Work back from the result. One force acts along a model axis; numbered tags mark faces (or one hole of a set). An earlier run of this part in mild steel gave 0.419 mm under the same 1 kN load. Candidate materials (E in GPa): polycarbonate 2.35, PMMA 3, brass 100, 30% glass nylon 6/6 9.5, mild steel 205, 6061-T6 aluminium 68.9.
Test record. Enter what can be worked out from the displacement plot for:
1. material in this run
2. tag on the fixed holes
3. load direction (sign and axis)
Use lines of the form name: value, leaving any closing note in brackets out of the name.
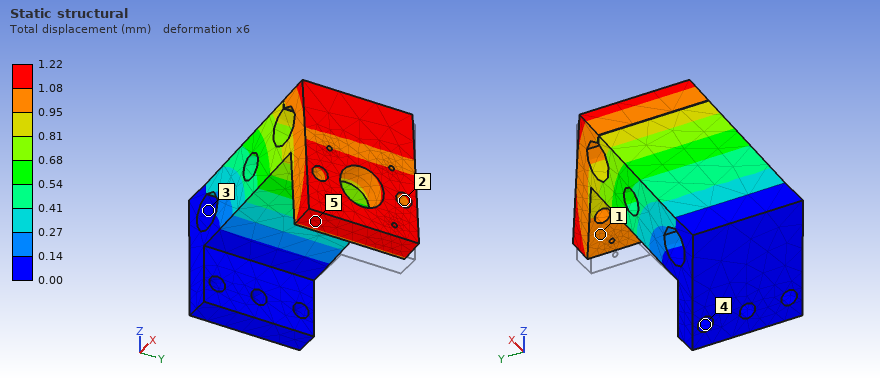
material in this run: 6061-T6 aluminium
tag on the fixed holes: 4
load direction: +Z
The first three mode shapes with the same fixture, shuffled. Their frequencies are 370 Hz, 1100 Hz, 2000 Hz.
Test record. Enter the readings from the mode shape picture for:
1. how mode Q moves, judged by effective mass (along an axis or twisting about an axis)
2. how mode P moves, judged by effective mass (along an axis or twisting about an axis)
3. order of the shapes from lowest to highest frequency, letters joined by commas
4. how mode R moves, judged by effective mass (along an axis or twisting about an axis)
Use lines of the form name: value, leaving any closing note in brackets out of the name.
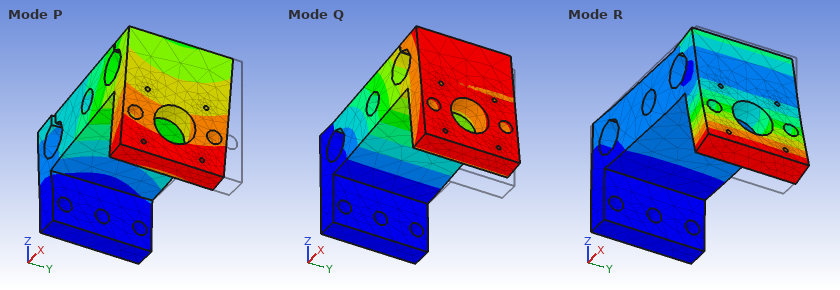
how mode Q moves, judged by effective mass: along Z
how mode P moves, judged by effective mass: along Y
order of the shapes from lowest to highest frequency, letters joined by commas: Q, P, R
how mode R moves, judged by effective mass: along X
